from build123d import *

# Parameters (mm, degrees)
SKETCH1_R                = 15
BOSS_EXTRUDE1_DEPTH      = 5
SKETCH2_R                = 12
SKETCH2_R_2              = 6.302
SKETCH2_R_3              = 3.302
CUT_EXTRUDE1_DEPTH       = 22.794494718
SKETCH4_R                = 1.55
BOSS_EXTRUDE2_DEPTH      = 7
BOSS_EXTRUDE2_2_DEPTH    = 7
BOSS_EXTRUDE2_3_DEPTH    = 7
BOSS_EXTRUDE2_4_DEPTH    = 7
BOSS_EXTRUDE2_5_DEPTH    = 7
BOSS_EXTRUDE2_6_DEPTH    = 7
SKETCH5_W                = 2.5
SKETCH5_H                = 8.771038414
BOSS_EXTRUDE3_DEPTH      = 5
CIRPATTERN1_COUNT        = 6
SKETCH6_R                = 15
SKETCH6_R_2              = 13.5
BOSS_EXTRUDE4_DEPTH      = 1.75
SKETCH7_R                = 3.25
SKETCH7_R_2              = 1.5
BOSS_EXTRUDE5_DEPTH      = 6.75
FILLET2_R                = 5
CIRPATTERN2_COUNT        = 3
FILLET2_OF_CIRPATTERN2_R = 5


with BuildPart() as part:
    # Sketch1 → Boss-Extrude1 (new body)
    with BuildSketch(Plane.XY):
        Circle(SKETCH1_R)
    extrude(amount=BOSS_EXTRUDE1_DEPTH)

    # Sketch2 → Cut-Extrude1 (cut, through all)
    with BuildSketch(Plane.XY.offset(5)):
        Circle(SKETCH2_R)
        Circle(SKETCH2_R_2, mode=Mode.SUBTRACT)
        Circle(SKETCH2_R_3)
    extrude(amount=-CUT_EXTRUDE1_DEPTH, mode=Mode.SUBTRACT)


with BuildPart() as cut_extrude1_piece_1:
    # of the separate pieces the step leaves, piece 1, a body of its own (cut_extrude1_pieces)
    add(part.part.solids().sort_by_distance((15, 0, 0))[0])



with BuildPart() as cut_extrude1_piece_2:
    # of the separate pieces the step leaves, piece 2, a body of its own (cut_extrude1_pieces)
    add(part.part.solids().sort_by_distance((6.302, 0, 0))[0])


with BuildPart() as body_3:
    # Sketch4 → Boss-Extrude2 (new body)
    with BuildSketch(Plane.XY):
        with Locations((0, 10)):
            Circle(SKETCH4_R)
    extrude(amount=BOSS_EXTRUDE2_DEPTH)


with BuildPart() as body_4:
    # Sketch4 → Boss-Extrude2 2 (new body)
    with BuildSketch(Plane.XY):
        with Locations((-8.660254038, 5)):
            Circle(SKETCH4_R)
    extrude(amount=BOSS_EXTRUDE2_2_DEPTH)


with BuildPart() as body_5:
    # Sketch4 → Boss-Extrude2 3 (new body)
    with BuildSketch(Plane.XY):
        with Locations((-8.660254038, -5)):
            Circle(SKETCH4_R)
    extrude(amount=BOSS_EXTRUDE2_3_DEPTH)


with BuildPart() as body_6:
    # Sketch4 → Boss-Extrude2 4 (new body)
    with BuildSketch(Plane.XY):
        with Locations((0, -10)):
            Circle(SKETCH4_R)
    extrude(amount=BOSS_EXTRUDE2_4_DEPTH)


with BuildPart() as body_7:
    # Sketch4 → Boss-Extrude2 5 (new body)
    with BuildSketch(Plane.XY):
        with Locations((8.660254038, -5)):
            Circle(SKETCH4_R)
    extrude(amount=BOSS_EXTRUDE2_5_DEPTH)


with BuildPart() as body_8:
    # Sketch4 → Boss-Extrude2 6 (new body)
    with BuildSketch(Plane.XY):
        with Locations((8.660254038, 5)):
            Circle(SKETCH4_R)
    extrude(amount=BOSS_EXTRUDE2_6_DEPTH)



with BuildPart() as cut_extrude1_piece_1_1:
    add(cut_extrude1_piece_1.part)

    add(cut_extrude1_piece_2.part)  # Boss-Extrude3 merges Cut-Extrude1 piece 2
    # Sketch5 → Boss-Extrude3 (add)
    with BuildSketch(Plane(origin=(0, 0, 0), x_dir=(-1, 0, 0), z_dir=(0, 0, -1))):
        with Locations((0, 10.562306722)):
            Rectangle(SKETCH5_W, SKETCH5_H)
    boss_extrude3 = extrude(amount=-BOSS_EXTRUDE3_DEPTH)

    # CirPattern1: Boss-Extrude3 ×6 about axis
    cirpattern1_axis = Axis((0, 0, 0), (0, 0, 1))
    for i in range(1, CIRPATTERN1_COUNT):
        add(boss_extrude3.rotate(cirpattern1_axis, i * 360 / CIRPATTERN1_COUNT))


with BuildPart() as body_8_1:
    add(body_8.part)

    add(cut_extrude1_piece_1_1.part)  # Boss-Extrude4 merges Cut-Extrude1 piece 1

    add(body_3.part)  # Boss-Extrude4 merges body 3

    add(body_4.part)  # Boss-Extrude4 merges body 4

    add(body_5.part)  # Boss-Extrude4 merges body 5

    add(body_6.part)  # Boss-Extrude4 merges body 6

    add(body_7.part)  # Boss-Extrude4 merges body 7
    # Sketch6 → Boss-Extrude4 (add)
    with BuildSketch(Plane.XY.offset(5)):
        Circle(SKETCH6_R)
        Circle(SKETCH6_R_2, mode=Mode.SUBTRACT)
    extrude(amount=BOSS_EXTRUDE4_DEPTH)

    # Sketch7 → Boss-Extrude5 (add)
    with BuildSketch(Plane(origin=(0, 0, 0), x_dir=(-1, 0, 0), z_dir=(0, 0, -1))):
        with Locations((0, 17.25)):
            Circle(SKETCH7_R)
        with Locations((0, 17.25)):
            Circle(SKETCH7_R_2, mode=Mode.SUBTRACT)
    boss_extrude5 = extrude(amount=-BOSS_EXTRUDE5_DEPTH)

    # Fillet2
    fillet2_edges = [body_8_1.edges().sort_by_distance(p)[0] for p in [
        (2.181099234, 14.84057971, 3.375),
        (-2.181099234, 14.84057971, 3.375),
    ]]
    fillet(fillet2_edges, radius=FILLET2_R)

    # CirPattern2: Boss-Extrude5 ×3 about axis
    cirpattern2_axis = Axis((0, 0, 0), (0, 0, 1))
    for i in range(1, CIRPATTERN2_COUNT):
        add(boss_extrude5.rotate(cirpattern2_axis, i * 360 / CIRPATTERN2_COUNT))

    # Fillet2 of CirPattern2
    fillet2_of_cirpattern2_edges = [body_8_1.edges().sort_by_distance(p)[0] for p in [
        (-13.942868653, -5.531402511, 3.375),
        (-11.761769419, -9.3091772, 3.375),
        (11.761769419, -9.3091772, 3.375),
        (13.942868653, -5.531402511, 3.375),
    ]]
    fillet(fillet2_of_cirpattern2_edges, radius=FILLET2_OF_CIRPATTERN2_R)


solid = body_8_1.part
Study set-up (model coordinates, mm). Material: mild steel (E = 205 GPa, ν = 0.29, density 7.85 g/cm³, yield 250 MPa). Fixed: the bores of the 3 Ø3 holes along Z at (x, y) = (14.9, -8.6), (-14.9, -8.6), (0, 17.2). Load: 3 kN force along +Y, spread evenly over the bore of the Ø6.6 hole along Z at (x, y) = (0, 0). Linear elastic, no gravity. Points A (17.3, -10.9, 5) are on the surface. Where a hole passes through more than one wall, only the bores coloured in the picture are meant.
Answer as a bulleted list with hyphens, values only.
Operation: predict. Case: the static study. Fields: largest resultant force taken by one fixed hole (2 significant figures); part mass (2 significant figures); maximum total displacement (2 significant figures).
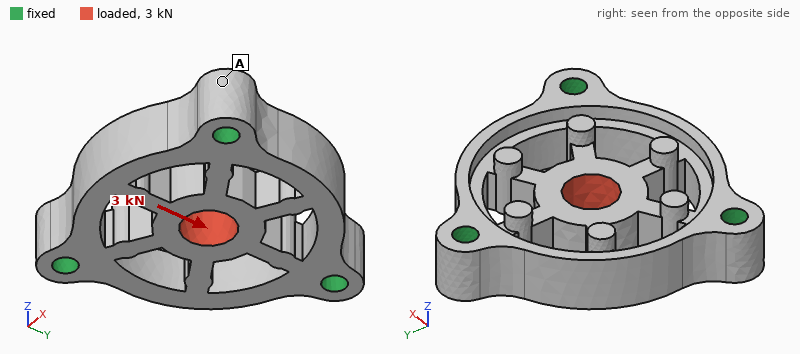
- 1.1 kN
- 24 g
- 7.8 µm
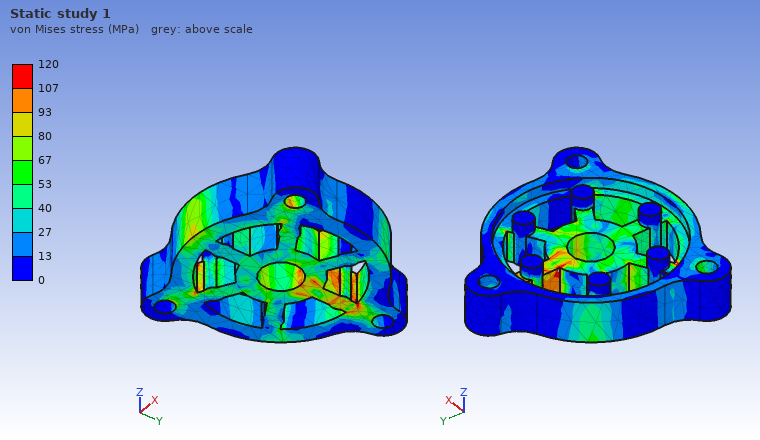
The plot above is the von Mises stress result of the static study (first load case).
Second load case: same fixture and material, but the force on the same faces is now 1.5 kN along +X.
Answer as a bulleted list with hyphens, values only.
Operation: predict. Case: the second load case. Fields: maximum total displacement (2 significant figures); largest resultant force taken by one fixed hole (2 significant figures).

- 3.8 µm
- 520 N
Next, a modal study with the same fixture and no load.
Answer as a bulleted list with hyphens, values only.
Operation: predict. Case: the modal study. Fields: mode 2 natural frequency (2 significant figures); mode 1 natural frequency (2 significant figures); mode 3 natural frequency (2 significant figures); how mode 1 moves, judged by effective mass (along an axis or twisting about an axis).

- 28 kHz
- 25 kHz
- 28 kHz
- along Z
